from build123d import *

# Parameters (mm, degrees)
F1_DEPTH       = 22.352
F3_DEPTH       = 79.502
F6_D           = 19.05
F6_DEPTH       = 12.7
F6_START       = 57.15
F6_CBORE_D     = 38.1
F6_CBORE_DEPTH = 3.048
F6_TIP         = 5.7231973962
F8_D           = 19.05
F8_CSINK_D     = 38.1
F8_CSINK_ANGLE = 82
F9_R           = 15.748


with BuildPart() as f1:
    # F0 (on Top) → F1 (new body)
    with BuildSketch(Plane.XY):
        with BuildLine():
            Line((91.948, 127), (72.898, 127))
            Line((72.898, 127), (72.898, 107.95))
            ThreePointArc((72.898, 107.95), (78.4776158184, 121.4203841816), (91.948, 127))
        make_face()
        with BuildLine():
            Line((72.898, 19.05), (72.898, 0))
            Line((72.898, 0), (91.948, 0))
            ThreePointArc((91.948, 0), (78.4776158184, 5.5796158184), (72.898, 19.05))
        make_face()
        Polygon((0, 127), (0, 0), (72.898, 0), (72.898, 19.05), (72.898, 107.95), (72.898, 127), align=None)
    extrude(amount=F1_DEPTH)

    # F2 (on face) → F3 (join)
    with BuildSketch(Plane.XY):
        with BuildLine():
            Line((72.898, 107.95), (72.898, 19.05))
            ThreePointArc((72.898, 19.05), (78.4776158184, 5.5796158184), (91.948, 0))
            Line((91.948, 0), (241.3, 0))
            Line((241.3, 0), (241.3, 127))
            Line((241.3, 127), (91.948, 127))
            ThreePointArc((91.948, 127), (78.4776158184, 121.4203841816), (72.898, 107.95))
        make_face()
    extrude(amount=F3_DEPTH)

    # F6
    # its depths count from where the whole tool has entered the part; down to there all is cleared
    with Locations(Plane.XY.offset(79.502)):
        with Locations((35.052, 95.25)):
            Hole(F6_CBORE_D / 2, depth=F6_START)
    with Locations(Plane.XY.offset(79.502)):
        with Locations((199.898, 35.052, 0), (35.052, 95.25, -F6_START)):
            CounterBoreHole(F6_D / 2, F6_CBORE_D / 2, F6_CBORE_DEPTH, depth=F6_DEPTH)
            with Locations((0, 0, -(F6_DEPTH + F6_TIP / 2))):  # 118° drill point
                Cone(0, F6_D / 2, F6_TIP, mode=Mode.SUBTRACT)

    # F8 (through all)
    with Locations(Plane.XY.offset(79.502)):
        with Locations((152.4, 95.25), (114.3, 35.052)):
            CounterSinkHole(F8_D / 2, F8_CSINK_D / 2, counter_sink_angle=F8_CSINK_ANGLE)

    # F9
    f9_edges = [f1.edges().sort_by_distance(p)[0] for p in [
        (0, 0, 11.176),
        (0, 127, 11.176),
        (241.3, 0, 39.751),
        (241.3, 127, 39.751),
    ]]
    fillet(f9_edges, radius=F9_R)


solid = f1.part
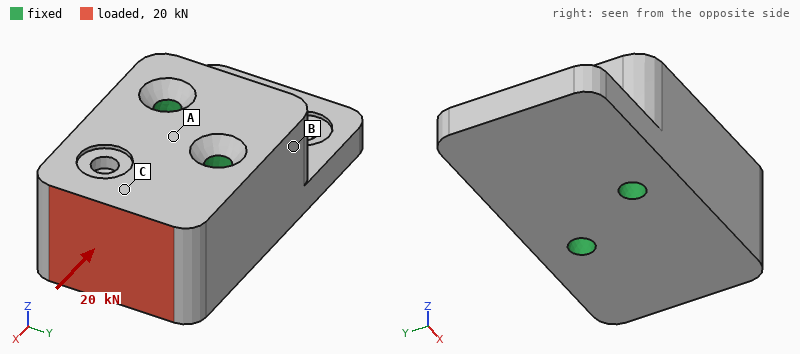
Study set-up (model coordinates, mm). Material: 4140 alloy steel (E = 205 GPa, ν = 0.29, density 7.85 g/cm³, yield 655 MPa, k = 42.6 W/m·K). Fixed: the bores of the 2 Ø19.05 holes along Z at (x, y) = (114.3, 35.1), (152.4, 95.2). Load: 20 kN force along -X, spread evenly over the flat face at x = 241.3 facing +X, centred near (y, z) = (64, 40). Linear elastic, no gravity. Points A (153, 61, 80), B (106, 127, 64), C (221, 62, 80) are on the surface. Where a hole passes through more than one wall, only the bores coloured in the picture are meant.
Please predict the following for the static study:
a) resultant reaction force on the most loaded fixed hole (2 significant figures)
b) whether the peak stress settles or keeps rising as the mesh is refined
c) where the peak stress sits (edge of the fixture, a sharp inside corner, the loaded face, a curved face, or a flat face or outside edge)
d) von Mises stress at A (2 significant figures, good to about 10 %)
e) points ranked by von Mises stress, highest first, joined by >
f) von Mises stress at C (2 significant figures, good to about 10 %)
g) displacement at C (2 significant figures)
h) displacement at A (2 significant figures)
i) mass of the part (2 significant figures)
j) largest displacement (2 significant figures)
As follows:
10 kN
keeps rising
edge of the fixture
1.8 MPa
C > A > B
2.9 MPa
1.4 µm
0.44 µm
14 kg
1.8 µm
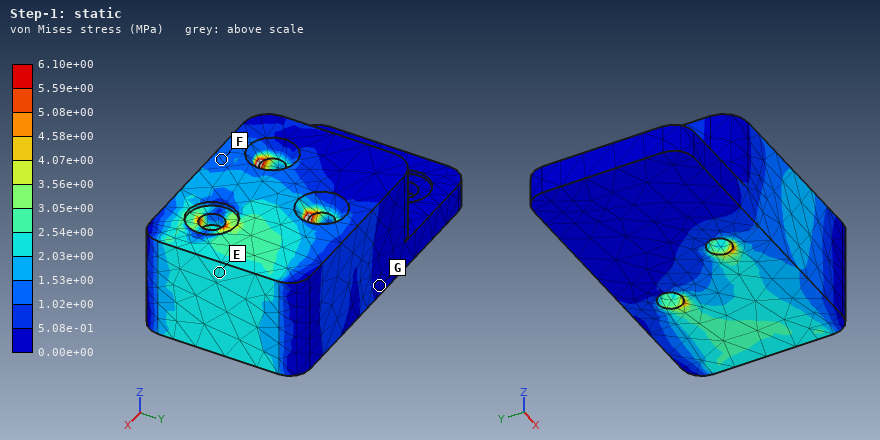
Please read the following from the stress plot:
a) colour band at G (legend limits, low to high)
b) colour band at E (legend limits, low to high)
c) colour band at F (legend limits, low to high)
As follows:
0.00e+00 to 5.08e-01 MPa
2.03e+00 to 2.54e+00 MPa
1.02e+00 to 1.53e+00 MPa
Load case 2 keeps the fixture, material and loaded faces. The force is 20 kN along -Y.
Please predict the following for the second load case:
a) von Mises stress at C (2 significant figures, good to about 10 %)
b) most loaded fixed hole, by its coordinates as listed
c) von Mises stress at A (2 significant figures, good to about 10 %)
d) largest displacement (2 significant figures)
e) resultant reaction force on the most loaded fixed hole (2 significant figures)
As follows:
4.9 MPa
(152.4, 95.2)
3.2 MPa
7.2 µm
31 kN
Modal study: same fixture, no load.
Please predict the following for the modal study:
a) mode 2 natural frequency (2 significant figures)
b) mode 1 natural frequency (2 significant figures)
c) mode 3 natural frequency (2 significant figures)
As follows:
4000 Hz
2400 Hz
4100 Hz
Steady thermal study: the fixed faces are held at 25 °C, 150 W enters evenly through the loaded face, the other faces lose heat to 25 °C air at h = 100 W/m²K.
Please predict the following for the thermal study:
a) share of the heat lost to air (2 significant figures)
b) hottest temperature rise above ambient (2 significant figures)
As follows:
38 %
31 K
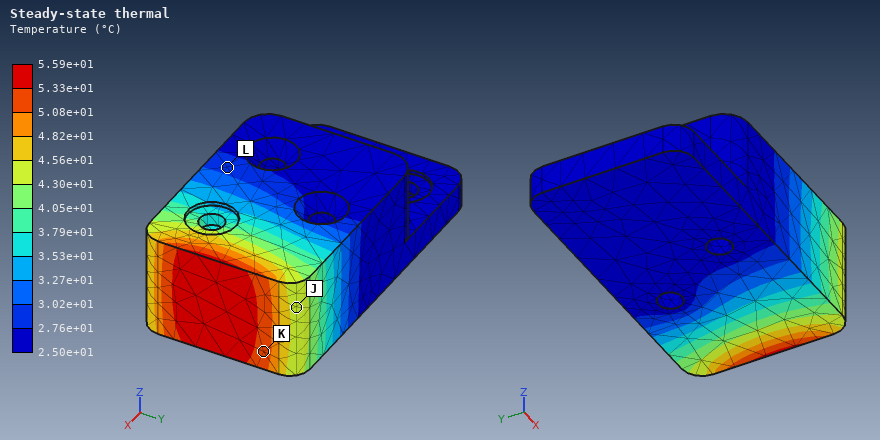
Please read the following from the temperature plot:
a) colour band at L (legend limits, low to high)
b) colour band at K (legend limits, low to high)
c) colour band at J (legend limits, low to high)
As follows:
2.76e+01 to 3.02e+01 °C
5.08e+01 to 5.33e+01 °C
4.30e+01 to 4.56e+01 °C
